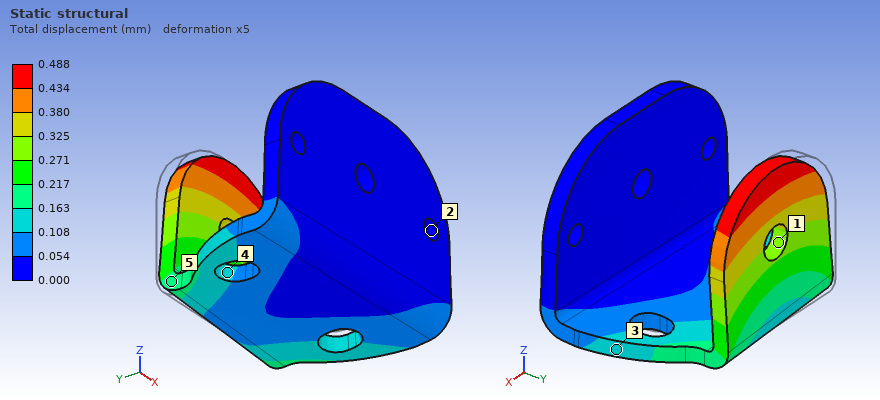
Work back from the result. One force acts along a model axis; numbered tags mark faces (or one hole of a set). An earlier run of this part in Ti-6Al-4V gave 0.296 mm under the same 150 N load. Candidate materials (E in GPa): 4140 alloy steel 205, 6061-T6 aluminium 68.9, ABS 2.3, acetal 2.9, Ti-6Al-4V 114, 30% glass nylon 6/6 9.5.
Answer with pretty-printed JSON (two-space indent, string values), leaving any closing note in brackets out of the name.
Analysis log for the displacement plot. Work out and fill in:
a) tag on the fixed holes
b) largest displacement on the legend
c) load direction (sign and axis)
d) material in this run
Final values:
{
  "tag on the fixed holes": "2",
  "largest displacement on the legend": "0.488 mm",
  "load direction": "+X",
  "material in this run": "6061-T6 aluminium"
}
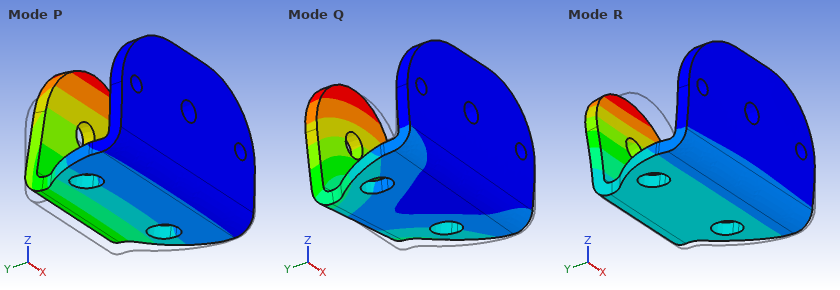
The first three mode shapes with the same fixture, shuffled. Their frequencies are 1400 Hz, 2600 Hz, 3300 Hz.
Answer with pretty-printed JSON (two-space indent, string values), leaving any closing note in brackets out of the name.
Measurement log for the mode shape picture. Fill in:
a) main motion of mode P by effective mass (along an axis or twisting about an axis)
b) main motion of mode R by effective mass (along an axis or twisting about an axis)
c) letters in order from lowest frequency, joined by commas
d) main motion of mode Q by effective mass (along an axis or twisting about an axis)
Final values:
{
  "main motion of mode P by effective mass": "along Z",
  "main motion of mode R by effective mass": "along Y",
  "letters in order from lowest frequency, joined by commas": "P, Q, R",
  "main motion of mode Q by effective mass": "along X"
}
